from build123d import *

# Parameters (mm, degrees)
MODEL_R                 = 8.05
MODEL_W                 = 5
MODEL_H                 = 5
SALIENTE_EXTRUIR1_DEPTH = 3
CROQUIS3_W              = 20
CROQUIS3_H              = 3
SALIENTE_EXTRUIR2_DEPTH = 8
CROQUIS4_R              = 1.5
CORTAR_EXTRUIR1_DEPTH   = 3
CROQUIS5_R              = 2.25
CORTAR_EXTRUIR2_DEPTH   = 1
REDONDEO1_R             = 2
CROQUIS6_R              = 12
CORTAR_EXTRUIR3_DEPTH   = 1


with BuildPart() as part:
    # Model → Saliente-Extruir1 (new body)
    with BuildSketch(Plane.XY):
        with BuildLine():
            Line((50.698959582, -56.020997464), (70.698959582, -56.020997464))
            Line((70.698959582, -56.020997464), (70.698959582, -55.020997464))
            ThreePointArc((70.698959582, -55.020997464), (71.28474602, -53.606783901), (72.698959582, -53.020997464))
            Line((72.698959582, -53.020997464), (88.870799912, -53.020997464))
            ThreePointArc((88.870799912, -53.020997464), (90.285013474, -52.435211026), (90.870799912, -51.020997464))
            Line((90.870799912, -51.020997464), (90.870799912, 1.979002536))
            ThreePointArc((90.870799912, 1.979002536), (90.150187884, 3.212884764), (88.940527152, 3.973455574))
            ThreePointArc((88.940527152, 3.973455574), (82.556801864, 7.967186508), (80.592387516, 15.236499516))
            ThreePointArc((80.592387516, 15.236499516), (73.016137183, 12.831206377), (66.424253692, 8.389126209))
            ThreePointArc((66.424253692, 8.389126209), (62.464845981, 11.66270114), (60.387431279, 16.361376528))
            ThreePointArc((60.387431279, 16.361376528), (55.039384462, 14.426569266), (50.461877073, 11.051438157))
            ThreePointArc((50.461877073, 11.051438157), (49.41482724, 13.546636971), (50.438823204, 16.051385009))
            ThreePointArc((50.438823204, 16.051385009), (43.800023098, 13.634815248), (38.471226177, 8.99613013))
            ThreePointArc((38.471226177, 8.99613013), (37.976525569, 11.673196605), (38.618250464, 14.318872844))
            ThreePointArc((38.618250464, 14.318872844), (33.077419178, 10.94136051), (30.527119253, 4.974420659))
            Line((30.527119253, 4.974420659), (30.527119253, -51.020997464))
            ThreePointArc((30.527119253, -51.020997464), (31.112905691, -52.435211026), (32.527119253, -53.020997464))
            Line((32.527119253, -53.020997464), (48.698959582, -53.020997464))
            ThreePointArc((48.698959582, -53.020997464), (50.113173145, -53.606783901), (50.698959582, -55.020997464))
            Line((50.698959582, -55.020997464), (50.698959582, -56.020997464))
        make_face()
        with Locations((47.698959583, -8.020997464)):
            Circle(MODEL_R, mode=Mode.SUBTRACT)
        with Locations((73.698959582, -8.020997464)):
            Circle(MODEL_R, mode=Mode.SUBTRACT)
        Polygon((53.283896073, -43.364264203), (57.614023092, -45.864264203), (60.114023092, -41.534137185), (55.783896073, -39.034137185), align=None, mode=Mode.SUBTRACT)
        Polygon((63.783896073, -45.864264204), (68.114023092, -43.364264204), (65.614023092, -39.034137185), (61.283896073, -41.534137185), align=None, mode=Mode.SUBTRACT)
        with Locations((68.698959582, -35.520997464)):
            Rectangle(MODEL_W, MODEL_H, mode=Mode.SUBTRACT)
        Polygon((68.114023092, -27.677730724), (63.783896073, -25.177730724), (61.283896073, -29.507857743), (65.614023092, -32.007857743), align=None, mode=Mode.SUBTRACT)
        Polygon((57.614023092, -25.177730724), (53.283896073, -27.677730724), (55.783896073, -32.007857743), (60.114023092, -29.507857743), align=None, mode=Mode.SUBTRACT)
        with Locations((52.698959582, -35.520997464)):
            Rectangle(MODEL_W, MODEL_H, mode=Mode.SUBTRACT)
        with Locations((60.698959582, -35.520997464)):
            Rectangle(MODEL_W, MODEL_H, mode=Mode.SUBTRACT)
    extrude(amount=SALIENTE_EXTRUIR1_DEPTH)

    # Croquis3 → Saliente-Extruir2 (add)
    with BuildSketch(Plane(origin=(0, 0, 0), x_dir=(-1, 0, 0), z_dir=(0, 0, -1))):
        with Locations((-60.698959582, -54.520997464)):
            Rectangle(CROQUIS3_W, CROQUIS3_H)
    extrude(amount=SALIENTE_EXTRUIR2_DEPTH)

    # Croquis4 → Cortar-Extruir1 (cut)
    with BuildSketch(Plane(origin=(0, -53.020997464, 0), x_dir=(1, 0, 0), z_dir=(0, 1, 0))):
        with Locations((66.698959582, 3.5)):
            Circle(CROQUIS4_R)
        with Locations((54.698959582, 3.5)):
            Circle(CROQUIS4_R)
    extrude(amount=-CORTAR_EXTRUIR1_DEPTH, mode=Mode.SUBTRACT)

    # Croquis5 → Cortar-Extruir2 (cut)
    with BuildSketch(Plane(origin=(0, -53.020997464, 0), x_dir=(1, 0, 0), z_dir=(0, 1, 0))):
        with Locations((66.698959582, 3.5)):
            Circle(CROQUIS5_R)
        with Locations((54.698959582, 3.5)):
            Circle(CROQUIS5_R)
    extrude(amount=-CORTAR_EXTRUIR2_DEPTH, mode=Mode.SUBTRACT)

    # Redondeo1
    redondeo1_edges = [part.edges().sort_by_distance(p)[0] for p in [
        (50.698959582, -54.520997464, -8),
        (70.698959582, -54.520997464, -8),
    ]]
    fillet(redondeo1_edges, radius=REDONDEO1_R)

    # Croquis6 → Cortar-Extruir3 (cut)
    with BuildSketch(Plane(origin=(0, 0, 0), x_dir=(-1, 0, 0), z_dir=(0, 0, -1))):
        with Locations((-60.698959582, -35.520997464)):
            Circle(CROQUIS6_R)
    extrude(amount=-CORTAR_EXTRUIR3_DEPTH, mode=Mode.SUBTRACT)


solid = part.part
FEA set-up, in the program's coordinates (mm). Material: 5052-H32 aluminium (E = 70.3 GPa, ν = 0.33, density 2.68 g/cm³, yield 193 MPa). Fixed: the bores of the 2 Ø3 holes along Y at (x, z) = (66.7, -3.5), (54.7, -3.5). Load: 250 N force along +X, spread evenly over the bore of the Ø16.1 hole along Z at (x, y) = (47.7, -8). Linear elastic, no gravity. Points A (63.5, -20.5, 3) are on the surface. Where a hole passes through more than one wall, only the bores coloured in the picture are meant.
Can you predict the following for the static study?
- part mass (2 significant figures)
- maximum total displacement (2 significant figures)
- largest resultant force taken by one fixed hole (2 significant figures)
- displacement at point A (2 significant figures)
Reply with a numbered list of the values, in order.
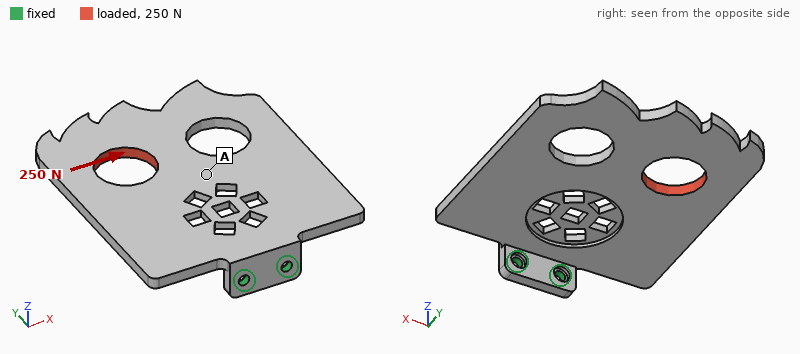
1. 28 g
2. 0.33 mm
3. 880 N
4. 0.14 mm
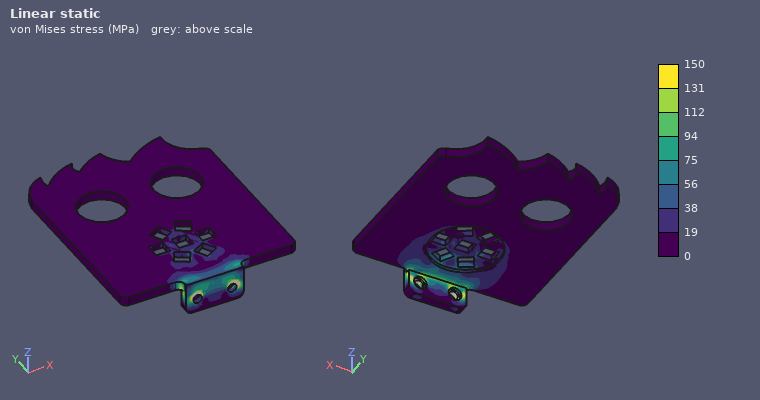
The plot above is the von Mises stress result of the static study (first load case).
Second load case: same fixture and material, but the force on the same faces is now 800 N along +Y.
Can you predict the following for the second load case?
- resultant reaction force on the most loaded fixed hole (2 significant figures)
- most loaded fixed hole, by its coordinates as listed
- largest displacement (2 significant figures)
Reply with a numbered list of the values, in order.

1. 1.2 kN
2. (54.7, -3.5)
3. 0.46 mm
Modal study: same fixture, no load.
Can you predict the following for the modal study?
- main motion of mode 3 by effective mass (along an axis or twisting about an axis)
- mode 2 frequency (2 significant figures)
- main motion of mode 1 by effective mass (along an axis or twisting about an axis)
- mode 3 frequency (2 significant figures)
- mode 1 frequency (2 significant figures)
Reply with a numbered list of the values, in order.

1. along X
2. 890 Hz
3. along Z
4. 1300 Hz
5. 340 Hz
